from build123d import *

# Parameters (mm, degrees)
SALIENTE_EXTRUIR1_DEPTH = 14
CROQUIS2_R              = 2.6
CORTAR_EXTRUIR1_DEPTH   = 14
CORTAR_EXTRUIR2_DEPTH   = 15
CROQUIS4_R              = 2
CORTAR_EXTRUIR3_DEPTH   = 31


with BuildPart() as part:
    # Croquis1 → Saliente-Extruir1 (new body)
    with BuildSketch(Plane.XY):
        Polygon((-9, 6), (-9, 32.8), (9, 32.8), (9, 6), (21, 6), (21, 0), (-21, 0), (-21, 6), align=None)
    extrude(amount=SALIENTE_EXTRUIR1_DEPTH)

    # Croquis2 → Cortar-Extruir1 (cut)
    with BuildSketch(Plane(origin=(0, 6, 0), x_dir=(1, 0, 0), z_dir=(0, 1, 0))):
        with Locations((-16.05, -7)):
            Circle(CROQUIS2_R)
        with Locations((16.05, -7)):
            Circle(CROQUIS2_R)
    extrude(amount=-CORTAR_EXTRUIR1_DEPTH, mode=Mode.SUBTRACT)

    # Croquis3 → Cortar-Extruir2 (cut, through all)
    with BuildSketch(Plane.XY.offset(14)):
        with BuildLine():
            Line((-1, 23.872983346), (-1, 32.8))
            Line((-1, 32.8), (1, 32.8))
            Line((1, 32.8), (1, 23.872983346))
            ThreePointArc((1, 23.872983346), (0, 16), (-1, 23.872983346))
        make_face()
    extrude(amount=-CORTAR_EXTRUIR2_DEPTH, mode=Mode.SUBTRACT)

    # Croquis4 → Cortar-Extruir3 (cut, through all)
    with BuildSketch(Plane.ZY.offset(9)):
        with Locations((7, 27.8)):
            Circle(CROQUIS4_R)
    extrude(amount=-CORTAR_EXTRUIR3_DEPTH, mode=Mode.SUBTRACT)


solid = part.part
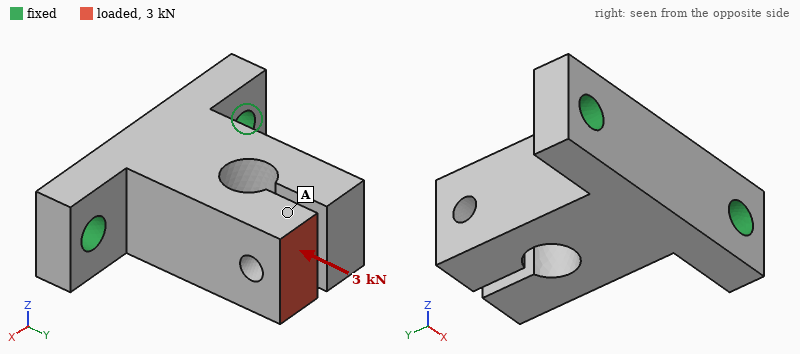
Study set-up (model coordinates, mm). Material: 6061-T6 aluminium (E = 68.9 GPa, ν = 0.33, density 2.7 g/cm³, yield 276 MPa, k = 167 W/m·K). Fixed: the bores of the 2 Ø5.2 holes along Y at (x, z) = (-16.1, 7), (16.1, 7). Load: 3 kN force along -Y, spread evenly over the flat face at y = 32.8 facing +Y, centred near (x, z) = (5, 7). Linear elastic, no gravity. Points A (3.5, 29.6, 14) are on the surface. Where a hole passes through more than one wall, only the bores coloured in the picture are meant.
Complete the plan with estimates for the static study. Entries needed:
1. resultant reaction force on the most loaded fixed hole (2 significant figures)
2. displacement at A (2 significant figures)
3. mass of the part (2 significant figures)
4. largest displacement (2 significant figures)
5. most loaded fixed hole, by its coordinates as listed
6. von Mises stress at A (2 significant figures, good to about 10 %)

2.2 kN
33 µm
24 g
44 µm
(16.1, 7)
20 MPa
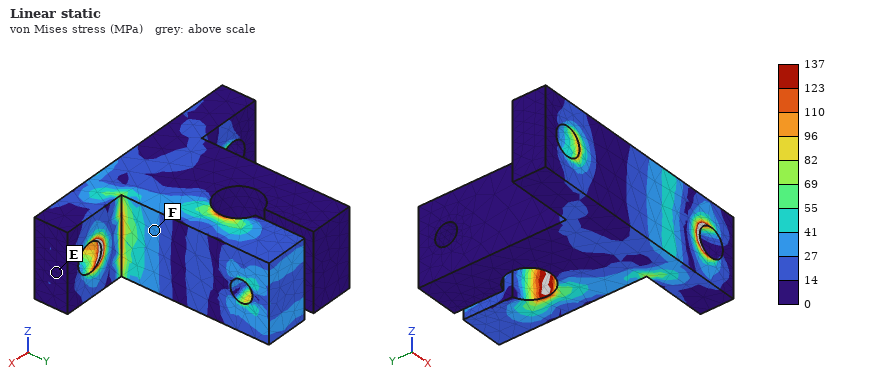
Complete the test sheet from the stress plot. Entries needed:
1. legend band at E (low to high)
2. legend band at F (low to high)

0 to 14 MPa
27 to 41 MPa
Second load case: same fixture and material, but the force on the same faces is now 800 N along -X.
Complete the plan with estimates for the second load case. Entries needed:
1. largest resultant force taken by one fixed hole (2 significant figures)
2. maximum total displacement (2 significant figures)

1.1 kN
0.17 mm
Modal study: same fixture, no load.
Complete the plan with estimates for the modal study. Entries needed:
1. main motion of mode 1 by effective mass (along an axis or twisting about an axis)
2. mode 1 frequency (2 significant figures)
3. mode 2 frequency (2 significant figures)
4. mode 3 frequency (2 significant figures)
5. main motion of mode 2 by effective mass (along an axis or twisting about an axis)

along Z
5100 Hz
8300 Hz
10 kHz
along X
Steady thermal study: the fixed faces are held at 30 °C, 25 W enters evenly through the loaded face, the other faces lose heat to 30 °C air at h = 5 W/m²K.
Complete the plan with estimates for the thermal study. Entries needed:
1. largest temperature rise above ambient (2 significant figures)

50 K
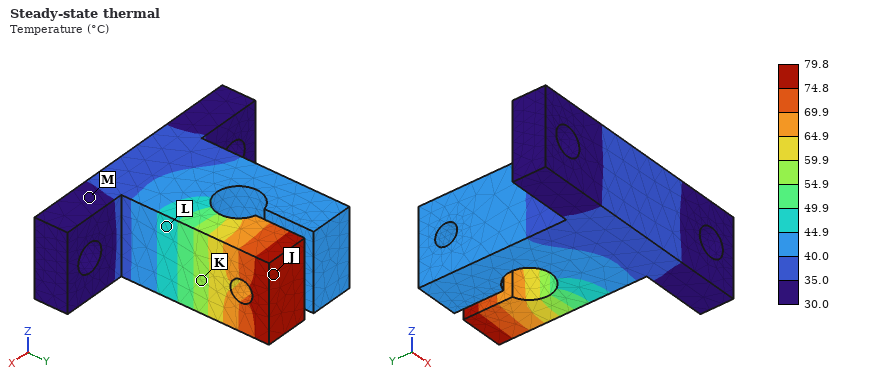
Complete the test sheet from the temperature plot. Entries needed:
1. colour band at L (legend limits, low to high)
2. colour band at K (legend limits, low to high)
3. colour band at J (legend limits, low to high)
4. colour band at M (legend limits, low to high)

44.9 to 49.9 °C
54.9 to 59.9 °C
74.8 to 79.8 °C
30.0 to 35.0 °C
